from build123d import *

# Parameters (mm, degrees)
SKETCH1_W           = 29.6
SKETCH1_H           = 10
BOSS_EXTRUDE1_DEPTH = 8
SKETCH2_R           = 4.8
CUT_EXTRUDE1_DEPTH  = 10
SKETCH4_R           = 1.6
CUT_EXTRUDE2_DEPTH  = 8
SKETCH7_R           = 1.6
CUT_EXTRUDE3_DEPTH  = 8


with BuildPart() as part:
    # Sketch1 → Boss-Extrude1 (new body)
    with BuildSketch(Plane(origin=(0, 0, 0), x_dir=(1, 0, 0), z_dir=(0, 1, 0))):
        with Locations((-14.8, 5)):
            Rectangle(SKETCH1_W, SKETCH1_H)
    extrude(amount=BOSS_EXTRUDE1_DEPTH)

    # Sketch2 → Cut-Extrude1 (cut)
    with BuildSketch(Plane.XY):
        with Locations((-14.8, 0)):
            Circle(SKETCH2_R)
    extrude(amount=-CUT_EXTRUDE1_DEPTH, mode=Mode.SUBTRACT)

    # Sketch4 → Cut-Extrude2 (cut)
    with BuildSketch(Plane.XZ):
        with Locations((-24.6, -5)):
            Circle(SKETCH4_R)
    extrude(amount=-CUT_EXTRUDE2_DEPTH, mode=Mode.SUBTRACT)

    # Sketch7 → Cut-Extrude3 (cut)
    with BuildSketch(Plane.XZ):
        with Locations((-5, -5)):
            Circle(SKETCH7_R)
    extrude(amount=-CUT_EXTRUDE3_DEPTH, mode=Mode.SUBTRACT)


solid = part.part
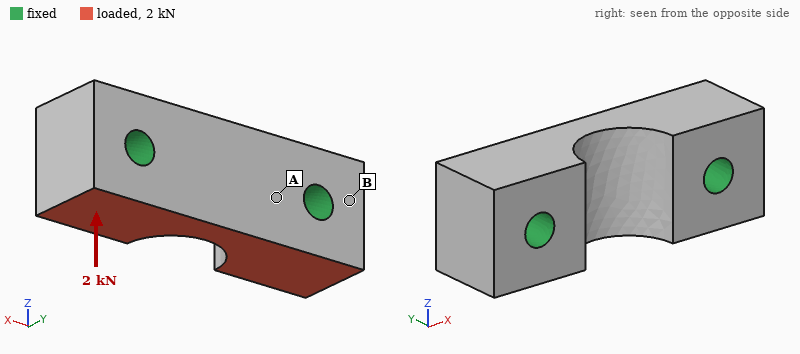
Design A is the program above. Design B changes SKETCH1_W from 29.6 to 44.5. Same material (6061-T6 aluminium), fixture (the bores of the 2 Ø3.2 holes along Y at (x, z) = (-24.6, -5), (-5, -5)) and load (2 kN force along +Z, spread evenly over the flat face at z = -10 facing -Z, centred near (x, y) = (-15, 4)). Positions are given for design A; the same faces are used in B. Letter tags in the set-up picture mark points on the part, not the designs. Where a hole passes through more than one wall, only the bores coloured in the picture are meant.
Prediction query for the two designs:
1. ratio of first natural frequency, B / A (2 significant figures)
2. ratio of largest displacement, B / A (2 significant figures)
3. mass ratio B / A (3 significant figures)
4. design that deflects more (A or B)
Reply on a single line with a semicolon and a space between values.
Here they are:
0.47; 2.7; 1.63; B
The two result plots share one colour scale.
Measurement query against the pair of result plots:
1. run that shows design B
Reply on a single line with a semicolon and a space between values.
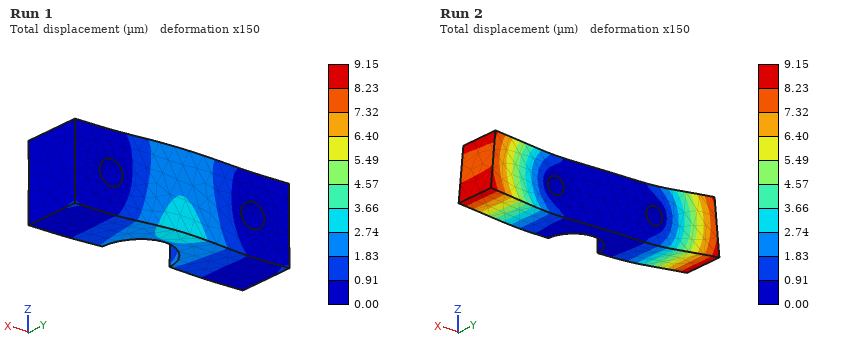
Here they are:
Run 2
